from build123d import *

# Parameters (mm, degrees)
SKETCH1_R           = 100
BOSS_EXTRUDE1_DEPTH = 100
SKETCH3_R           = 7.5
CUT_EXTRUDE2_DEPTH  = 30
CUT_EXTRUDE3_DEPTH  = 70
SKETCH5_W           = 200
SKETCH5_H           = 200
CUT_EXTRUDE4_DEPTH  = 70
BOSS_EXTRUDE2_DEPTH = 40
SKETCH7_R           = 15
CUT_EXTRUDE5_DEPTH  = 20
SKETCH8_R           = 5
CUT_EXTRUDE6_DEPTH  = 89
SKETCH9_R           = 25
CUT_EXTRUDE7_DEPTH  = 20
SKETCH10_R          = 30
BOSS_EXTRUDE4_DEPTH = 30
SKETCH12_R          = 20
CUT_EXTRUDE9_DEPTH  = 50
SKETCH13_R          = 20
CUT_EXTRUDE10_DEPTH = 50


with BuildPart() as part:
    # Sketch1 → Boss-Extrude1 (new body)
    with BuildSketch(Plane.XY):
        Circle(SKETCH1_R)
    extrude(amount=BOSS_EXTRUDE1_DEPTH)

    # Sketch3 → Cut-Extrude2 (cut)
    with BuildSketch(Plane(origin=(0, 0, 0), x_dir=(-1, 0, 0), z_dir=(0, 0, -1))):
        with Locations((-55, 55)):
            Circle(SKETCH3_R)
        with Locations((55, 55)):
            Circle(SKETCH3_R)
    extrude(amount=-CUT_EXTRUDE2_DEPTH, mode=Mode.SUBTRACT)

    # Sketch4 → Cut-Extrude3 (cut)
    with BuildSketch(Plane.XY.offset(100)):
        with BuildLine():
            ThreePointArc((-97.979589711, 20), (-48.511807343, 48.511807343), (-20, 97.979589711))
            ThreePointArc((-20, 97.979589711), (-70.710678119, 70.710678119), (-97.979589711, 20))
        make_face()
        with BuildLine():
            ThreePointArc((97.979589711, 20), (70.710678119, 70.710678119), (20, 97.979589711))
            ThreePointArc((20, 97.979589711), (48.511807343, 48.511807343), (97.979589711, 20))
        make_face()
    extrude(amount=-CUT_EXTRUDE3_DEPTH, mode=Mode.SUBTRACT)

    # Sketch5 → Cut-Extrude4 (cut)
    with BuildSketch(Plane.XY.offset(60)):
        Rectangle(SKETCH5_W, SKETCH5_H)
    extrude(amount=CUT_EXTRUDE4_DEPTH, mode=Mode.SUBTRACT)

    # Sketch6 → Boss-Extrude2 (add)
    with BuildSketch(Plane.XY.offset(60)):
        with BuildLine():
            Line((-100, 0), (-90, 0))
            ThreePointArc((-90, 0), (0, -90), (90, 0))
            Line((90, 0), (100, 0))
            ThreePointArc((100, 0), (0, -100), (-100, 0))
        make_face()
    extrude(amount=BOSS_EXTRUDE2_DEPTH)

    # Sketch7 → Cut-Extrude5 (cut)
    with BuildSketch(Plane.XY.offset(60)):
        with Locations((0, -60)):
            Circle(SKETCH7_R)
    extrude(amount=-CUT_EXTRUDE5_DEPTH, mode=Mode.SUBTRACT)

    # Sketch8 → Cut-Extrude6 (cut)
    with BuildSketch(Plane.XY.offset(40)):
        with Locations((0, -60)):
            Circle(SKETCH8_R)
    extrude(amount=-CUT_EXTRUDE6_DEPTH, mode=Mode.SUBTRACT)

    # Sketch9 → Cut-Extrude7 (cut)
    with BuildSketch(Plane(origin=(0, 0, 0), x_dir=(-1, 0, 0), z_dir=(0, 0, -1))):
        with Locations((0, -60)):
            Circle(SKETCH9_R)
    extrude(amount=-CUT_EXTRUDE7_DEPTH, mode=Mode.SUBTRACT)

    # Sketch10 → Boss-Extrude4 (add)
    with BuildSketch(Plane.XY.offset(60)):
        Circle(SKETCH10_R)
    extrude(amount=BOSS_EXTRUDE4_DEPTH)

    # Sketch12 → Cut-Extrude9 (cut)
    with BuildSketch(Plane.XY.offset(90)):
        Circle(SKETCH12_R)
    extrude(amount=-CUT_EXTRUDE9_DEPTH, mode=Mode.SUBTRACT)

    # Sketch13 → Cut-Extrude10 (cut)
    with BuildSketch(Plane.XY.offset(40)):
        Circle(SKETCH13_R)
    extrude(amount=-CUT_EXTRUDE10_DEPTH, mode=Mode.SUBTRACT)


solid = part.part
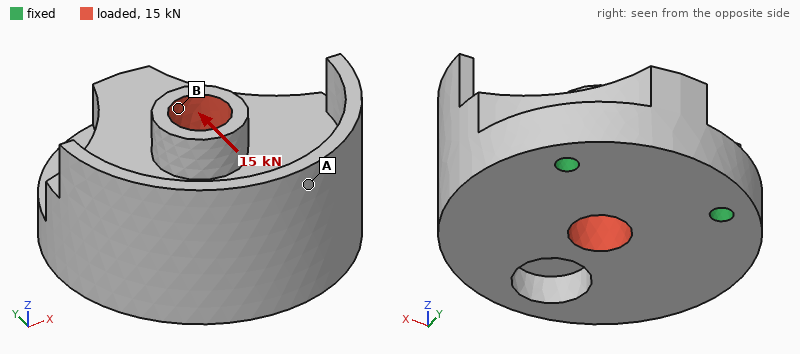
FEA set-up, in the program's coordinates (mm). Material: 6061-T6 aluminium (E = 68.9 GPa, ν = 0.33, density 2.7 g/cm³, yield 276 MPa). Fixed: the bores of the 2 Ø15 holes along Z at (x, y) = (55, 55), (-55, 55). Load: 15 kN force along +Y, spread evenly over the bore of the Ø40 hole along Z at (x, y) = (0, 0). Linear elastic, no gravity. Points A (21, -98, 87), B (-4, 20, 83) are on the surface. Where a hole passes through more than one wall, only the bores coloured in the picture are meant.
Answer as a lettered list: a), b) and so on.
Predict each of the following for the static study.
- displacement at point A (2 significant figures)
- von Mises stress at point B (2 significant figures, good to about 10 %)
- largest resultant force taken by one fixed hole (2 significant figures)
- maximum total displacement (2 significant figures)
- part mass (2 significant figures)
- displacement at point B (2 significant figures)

a) 75 µm
b) 5.3 MPa
c) 7.5 kN
d) 80 µm
e) 4.8 kg
f) 39 µm
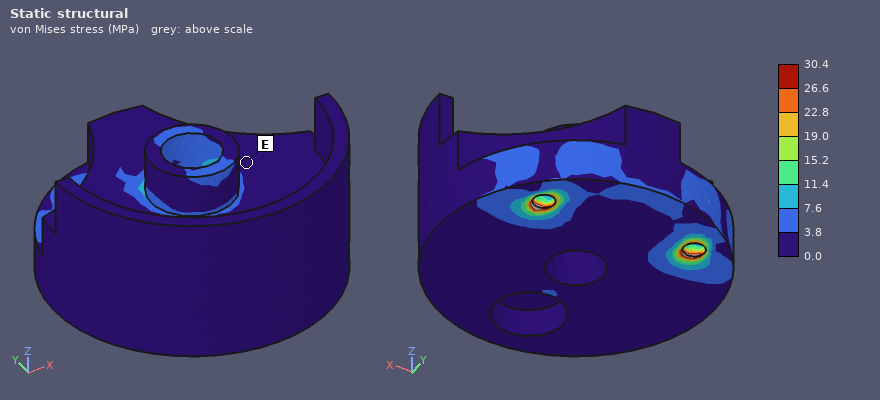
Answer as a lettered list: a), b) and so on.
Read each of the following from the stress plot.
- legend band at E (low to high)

a) 0.0 to 3.8 MPa
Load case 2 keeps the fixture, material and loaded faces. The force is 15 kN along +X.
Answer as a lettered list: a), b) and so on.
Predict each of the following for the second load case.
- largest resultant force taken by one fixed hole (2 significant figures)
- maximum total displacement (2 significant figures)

a) 11 kN
b) 17 µm
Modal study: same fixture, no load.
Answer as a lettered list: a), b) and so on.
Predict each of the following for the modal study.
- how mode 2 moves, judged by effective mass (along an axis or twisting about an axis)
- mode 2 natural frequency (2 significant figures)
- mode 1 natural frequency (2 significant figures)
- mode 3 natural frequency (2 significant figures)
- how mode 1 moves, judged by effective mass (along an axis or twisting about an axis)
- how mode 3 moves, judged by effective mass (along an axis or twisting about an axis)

a) along X
b) 2400 Hz
c) 870 Hz
d) 2600 Hz
e) along Z
f) along X
